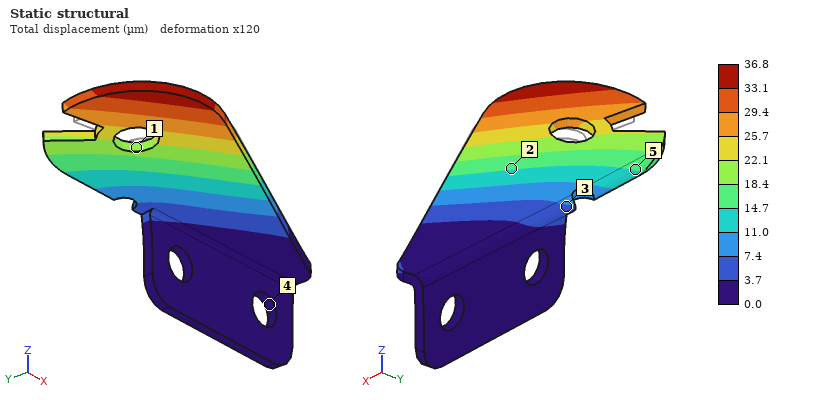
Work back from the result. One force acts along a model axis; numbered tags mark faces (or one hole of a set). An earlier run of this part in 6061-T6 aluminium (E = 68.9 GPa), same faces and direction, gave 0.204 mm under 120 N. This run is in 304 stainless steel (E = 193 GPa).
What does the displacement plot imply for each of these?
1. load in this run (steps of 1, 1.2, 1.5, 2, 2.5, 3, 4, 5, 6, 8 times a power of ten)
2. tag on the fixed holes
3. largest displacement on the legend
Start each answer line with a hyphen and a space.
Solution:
- 60 N
- 4
- 36.8 µm
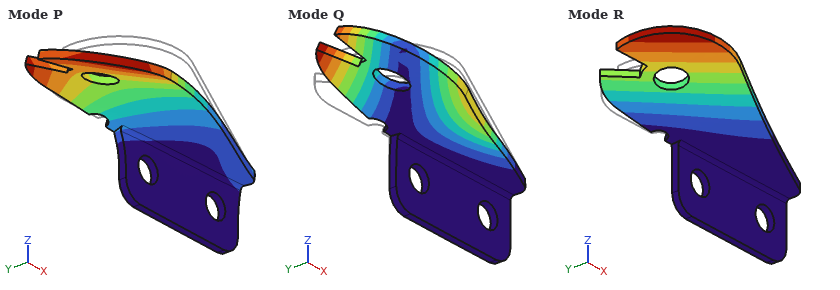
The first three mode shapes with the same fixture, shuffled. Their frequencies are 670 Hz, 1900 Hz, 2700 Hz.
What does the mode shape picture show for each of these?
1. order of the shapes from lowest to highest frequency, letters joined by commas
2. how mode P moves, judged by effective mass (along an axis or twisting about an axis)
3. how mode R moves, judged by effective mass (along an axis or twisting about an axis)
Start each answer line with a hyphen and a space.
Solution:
- R, Q, P
- along Y
- along Z
